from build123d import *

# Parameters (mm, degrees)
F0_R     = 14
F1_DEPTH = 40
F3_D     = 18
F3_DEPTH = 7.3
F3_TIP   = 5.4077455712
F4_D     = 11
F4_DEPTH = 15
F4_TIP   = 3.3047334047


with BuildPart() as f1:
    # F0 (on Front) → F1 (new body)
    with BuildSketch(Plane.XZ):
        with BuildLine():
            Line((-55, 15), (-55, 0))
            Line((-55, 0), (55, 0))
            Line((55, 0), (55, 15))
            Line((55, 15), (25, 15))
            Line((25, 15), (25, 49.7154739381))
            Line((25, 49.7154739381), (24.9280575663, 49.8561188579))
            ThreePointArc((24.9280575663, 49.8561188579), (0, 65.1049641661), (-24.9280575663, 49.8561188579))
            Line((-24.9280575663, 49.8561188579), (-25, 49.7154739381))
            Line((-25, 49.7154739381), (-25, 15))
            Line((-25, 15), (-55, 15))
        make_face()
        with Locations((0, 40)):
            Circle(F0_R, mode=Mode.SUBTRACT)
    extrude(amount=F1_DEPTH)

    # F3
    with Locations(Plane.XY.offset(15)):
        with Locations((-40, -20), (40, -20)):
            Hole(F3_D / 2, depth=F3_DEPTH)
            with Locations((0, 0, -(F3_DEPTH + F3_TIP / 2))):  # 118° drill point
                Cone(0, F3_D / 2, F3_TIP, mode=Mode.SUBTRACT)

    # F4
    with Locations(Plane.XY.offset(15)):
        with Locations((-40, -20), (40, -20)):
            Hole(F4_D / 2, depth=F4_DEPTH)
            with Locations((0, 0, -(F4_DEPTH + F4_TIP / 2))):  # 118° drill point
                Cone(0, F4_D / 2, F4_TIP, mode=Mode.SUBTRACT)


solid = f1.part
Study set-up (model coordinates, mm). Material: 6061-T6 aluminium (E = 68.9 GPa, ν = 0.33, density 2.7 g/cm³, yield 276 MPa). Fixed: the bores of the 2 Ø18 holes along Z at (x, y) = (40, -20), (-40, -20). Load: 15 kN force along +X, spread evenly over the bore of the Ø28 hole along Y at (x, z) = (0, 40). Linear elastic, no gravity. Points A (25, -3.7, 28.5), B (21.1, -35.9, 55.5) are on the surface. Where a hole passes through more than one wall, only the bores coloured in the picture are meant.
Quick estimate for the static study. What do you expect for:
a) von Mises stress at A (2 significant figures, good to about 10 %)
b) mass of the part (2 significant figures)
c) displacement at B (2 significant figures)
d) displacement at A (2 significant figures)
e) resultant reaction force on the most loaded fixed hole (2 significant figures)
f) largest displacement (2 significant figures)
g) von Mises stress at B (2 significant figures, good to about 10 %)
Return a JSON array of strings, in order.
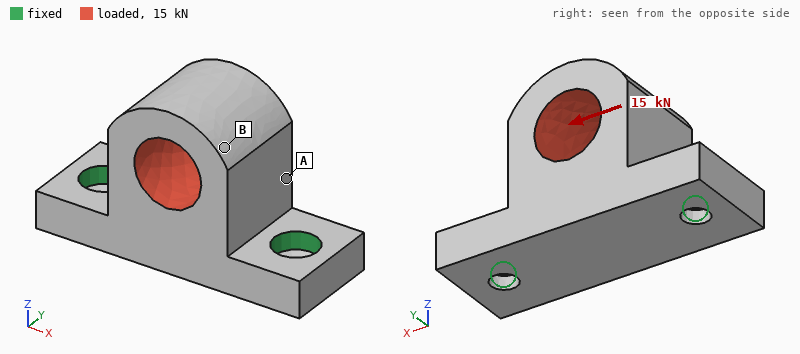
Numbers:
["31 MPa", "340 g", "68 µm", "28 µm", "11 kN", "70 µm", "19 MPa"]
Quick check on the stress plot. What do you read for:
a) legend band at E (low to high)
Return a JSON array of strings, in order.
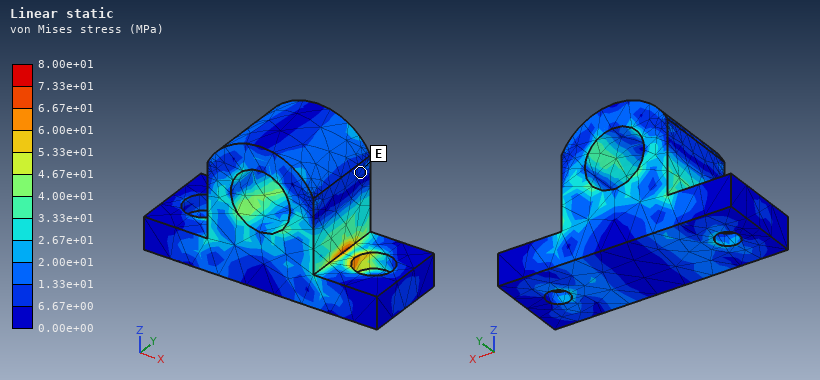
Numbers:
["6.67e+00 to 1.33e+01 MPa"]
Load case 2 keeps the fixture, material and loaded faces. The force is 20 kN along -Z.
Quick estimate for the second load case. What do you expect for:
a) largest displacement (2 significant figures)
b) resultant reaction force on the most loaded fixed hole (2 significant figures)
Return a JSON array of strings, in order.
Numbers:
["33 µm", "10 kN"]
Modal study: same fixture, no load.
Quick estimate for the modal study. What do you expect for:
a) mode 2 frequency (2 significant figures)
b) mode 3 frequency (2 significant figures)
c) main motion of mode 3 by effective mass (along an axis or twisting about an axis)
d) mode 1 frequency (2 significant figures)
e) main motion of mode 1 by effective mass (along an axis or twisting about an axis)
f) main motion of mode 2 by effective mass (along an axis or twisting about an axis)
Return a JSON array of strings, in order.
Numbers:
["6500 Hz", "8700 Hz", "along Z", "3400 Hz", "along Y", "along X"]
